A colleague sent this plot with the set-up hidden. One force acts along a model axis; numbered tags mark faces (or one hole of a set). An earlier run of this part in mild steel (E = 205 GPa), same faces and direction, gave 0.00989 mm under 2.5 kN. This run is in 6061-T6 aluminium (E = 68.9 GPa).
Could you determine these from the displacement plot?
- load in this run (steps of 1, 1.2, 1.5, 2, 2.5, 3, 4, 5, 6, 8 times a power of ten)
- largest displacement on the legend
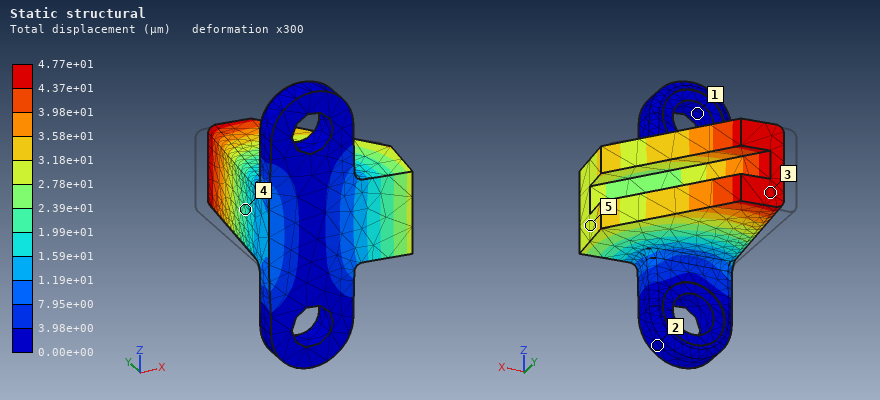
4 kN
4.77e+01 µm
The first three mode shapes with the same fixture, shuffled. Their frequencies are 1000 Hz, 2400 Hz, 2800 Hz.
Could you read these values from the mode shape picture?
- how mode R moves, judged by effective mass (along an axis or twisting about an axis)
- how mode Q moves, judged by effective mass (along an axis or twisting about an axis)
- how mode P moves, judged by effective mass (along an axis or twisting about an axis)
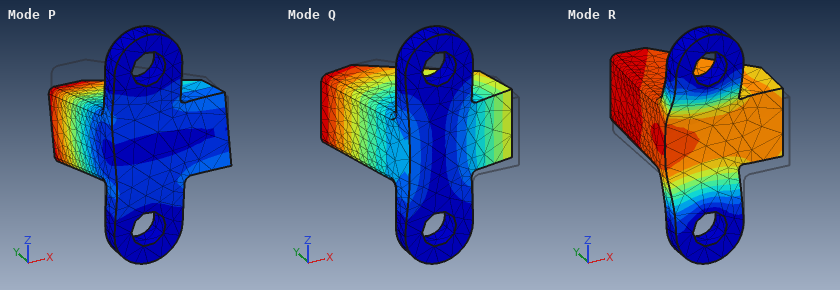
along Y
along X
along Z
